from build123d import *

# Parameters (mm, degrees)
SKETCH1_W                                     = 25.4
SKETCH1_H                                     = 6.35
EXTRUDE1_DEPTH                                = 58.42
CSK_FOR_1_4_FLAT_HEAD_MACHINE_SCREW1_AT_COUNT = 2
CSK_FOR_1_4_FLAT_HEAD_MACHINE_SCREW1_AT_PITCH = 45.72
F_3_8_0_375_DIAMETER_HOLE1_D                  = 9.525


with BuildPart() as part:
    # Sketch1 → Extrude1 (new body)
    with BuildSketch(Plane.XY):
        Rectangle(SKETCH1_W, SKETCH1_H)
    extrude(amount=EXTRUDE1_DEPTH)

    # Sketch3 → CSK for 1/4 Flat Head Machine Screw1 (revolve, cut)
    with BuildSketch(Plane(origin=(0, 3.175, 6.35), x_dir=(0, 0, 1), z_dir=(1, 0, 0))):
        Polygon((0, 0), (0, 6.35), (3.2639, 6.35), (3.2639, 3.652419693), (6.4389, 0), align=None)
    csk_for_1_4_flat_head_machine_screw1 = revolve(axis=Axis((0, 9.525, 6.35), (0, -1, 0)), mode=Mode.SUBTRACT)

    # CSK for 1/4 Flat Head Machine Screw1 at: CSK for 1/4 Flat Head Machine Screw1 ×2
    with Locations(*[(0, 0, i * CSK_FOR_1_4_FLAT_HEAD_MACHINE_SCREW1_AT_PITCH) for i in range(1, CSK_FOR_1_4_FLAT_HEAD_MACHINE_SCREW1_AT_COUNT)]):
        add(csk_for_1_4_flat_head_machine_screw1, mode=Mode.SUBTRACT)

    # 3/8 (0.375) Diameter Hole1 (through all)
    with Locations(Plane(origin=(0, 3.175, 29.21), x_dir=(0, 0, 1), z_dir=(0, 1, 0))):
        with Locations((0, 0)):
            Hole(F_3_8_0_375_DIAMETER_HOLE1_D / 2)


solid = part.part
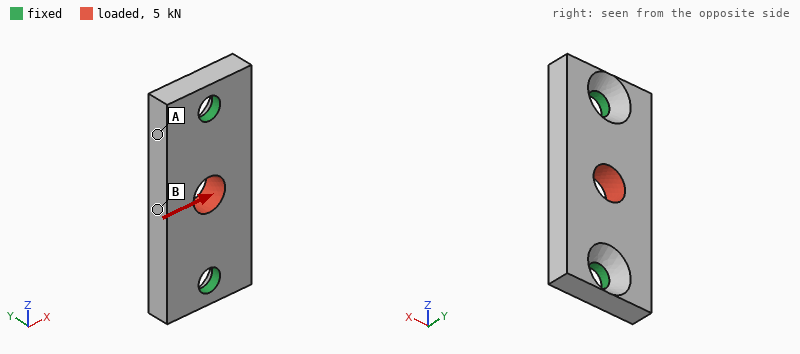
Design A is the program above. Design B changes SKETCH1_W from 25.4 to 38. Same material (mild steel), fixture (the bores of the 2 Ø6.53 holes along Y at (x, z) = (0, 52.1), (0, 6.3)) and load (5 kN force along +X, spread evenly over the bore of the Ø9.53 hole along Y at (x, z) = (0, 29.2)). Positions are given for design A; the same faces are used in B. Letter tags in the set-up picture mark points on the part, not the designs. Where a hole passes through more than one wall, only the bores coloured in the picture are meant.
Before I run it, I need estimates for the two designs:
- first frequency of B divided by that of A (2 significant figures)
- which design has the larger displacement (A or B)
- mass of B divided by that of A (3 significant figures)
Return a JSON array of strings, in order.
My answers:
["0.56", "A", "1.57"]
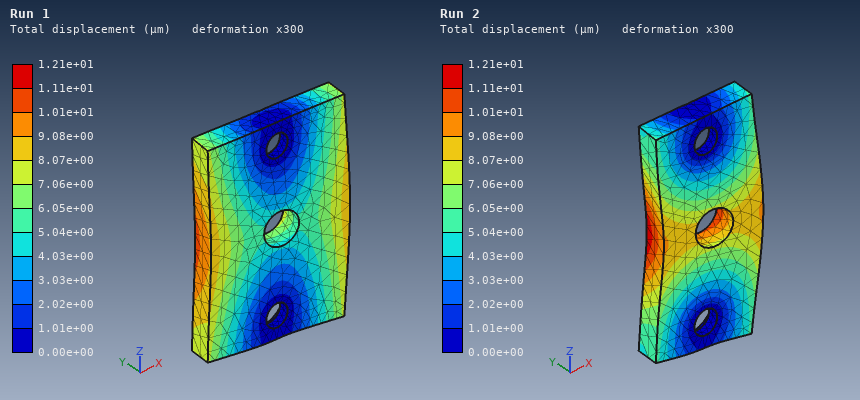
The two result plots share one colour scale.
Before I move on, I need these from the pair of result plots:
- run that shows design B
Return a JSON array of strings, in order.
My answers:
["Run 1"]
